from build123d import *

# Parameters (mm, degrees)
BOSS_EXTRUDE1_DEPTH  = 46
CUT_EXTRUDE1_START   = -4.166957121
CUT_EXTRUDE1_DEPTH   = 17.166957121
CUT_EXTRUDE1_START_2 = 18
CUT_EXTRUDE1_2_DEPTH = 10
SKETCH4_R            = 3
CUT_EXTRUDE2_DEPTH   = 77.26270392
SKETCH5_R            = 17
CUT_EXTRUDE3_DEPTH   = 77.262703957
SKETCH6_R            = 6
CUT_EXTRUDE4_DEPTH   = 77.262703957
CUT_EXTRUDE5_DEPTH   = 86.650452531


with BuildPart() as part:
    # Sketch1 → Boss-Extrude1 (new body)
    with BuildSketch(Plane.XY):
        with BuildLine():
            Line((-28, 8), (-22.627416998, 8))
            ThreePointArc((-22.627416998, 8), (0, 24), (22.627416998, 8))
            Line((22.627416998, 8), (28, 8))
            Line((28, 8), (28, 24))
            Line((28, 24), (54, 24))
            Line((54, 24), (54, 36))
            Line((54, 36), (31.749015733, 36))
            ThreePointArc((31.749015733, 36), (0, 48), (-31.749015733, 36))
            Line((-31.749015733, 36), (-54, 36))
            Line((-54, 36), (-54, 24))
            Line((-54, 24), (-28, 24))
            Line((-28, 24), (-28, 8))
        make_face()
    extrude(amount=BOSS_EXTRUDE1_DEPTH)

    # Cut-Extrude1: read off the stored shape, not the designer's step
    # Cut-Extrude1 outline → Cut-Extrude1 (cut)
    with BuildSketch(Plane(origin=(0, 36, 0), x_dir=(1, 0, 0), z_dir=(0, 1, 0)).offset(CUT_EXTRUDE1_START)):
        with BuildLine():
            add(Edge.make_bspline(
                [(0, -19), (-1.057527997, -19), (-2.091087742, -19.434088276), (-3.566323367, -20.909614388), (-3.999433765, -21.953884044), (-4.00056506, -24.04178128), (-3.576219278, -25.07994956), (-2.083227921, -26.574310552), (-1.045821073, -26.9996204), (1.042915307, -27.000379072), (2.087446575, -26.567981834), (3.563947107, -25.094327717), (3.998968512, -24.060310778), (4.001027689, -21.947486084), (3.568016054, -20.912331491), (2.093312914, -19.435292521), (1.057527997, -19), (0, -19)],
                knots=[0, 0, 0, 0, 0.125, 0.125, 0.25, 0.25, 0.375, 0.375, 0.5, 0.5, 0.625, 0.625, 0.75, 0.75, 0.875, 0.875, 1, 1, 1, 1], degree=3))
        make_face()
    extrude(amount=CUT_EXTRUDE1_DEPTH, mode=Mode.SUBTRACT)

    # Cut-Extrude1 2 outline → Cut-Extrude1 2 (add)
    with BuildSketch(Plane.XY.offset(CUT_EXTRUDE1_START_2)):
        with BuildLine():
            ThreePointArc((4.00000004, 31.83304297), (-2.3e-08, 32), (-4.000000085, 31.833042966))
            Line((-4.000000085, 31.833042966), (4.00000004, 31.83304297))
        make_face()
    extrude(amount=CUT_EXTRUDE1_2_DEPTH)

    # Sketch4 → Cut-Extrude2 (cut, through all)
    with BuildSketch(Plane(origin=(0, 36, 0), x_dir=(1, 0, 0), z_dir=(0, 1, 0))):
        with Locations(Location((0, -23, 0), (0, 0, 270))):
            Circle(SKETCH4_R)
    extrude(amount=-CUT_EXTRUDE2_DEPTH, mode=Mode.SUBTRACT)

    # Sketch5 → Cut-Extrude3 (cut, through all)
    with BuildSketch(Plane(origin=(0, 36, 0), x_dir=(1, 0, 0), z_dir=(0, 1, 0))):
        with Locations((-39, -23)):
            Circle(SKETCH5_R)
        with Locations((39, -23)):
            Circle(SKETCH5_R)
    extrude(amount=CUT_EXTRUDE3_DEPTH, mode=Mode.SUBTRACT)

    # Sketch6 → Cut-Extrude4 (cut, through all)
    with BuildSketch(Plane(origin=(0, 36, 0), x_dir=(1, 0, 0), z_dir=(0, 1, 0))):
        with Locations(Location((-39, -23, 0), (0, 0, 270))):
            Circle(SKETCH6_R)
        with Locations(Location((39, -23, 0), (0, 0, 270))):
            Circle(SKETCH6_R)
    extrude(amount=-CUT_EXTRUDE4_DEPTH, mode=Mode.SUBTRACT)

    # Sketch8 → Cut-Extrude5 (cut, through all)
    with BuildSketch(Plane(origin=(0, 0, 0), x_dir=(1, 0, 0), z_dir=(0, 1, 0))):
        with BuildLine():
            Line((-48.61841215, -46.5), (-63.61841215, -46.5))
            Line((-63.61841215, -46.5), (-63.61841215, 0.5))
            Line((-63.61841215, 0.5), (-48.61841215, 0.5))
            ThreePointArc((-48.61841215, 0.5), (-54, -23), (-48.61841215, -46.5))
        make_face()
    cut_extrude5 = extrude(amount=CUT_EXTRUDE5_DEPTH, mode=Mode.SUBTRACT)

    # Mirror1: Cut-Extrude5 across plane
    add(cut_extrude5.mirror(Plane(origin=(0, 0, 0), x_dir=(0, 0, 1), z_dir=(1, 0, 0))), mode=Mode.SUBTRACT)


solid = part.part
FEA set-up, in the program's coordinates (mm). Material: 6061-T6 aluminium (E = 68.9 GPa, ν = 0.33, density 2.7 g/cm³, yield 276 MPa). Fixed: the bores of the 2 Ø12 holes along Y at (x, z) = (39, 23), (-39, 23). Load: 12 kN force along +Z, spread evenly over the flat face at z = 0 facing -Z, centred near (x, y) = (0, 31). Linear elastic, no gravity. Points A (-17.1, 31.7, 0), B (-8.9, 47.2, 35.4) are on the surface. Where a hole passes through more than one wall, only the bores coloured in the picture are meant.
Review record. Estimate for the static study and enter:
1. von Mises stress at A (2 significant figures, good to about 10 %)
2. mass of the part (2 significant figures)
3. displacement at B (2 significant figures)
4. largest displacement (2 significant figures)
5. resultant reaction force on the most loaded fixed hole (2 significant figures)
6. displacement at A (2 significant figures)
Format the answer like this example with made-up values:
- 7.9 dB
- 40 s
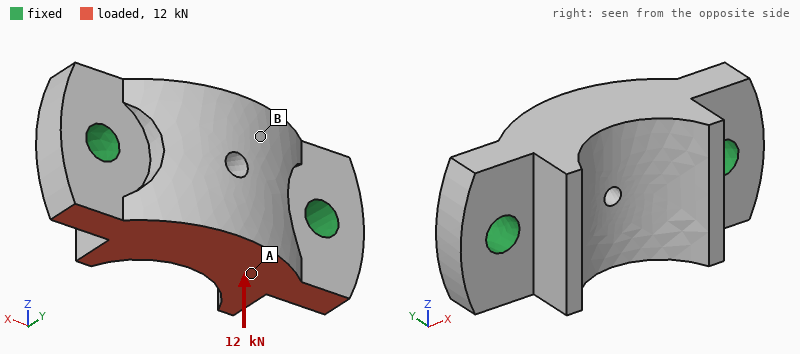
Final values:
- 13 MPa
- 250 g
- 12 µm
- 16 µm
- 6.0 kN
- 10 µm
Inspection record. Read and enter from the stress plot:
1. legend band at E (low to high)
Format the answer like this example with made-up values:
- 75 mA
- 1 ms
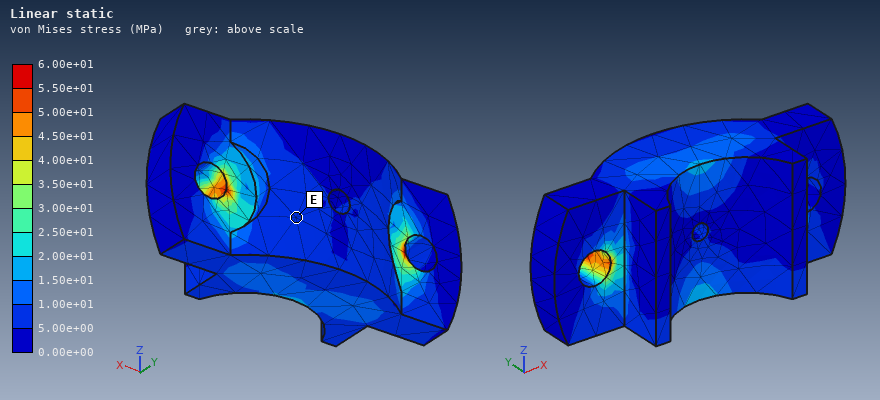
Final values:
- 5.00e+00 to 1.00e+01 MPa
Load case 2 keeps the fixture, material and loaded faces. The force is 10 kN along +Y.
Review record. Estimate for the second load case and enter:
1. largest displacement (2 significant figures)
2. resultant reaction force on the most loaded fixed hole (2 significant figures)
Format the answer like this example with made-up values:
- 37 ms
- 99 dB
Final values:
- 72 µm
- 5.1 kN
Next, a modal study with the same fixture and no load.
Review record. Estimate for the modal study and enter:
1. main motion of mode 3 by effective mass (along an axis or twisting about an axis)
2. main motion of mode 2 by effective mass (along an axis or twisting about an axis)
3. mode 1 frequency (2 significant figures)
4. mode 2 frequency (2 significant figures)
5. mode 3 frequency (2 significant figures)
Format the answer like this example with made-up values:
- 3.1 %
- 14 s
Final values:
- along Z
- along Y
- 7400 Hz
- 9100 Hz
- 12 kHz
